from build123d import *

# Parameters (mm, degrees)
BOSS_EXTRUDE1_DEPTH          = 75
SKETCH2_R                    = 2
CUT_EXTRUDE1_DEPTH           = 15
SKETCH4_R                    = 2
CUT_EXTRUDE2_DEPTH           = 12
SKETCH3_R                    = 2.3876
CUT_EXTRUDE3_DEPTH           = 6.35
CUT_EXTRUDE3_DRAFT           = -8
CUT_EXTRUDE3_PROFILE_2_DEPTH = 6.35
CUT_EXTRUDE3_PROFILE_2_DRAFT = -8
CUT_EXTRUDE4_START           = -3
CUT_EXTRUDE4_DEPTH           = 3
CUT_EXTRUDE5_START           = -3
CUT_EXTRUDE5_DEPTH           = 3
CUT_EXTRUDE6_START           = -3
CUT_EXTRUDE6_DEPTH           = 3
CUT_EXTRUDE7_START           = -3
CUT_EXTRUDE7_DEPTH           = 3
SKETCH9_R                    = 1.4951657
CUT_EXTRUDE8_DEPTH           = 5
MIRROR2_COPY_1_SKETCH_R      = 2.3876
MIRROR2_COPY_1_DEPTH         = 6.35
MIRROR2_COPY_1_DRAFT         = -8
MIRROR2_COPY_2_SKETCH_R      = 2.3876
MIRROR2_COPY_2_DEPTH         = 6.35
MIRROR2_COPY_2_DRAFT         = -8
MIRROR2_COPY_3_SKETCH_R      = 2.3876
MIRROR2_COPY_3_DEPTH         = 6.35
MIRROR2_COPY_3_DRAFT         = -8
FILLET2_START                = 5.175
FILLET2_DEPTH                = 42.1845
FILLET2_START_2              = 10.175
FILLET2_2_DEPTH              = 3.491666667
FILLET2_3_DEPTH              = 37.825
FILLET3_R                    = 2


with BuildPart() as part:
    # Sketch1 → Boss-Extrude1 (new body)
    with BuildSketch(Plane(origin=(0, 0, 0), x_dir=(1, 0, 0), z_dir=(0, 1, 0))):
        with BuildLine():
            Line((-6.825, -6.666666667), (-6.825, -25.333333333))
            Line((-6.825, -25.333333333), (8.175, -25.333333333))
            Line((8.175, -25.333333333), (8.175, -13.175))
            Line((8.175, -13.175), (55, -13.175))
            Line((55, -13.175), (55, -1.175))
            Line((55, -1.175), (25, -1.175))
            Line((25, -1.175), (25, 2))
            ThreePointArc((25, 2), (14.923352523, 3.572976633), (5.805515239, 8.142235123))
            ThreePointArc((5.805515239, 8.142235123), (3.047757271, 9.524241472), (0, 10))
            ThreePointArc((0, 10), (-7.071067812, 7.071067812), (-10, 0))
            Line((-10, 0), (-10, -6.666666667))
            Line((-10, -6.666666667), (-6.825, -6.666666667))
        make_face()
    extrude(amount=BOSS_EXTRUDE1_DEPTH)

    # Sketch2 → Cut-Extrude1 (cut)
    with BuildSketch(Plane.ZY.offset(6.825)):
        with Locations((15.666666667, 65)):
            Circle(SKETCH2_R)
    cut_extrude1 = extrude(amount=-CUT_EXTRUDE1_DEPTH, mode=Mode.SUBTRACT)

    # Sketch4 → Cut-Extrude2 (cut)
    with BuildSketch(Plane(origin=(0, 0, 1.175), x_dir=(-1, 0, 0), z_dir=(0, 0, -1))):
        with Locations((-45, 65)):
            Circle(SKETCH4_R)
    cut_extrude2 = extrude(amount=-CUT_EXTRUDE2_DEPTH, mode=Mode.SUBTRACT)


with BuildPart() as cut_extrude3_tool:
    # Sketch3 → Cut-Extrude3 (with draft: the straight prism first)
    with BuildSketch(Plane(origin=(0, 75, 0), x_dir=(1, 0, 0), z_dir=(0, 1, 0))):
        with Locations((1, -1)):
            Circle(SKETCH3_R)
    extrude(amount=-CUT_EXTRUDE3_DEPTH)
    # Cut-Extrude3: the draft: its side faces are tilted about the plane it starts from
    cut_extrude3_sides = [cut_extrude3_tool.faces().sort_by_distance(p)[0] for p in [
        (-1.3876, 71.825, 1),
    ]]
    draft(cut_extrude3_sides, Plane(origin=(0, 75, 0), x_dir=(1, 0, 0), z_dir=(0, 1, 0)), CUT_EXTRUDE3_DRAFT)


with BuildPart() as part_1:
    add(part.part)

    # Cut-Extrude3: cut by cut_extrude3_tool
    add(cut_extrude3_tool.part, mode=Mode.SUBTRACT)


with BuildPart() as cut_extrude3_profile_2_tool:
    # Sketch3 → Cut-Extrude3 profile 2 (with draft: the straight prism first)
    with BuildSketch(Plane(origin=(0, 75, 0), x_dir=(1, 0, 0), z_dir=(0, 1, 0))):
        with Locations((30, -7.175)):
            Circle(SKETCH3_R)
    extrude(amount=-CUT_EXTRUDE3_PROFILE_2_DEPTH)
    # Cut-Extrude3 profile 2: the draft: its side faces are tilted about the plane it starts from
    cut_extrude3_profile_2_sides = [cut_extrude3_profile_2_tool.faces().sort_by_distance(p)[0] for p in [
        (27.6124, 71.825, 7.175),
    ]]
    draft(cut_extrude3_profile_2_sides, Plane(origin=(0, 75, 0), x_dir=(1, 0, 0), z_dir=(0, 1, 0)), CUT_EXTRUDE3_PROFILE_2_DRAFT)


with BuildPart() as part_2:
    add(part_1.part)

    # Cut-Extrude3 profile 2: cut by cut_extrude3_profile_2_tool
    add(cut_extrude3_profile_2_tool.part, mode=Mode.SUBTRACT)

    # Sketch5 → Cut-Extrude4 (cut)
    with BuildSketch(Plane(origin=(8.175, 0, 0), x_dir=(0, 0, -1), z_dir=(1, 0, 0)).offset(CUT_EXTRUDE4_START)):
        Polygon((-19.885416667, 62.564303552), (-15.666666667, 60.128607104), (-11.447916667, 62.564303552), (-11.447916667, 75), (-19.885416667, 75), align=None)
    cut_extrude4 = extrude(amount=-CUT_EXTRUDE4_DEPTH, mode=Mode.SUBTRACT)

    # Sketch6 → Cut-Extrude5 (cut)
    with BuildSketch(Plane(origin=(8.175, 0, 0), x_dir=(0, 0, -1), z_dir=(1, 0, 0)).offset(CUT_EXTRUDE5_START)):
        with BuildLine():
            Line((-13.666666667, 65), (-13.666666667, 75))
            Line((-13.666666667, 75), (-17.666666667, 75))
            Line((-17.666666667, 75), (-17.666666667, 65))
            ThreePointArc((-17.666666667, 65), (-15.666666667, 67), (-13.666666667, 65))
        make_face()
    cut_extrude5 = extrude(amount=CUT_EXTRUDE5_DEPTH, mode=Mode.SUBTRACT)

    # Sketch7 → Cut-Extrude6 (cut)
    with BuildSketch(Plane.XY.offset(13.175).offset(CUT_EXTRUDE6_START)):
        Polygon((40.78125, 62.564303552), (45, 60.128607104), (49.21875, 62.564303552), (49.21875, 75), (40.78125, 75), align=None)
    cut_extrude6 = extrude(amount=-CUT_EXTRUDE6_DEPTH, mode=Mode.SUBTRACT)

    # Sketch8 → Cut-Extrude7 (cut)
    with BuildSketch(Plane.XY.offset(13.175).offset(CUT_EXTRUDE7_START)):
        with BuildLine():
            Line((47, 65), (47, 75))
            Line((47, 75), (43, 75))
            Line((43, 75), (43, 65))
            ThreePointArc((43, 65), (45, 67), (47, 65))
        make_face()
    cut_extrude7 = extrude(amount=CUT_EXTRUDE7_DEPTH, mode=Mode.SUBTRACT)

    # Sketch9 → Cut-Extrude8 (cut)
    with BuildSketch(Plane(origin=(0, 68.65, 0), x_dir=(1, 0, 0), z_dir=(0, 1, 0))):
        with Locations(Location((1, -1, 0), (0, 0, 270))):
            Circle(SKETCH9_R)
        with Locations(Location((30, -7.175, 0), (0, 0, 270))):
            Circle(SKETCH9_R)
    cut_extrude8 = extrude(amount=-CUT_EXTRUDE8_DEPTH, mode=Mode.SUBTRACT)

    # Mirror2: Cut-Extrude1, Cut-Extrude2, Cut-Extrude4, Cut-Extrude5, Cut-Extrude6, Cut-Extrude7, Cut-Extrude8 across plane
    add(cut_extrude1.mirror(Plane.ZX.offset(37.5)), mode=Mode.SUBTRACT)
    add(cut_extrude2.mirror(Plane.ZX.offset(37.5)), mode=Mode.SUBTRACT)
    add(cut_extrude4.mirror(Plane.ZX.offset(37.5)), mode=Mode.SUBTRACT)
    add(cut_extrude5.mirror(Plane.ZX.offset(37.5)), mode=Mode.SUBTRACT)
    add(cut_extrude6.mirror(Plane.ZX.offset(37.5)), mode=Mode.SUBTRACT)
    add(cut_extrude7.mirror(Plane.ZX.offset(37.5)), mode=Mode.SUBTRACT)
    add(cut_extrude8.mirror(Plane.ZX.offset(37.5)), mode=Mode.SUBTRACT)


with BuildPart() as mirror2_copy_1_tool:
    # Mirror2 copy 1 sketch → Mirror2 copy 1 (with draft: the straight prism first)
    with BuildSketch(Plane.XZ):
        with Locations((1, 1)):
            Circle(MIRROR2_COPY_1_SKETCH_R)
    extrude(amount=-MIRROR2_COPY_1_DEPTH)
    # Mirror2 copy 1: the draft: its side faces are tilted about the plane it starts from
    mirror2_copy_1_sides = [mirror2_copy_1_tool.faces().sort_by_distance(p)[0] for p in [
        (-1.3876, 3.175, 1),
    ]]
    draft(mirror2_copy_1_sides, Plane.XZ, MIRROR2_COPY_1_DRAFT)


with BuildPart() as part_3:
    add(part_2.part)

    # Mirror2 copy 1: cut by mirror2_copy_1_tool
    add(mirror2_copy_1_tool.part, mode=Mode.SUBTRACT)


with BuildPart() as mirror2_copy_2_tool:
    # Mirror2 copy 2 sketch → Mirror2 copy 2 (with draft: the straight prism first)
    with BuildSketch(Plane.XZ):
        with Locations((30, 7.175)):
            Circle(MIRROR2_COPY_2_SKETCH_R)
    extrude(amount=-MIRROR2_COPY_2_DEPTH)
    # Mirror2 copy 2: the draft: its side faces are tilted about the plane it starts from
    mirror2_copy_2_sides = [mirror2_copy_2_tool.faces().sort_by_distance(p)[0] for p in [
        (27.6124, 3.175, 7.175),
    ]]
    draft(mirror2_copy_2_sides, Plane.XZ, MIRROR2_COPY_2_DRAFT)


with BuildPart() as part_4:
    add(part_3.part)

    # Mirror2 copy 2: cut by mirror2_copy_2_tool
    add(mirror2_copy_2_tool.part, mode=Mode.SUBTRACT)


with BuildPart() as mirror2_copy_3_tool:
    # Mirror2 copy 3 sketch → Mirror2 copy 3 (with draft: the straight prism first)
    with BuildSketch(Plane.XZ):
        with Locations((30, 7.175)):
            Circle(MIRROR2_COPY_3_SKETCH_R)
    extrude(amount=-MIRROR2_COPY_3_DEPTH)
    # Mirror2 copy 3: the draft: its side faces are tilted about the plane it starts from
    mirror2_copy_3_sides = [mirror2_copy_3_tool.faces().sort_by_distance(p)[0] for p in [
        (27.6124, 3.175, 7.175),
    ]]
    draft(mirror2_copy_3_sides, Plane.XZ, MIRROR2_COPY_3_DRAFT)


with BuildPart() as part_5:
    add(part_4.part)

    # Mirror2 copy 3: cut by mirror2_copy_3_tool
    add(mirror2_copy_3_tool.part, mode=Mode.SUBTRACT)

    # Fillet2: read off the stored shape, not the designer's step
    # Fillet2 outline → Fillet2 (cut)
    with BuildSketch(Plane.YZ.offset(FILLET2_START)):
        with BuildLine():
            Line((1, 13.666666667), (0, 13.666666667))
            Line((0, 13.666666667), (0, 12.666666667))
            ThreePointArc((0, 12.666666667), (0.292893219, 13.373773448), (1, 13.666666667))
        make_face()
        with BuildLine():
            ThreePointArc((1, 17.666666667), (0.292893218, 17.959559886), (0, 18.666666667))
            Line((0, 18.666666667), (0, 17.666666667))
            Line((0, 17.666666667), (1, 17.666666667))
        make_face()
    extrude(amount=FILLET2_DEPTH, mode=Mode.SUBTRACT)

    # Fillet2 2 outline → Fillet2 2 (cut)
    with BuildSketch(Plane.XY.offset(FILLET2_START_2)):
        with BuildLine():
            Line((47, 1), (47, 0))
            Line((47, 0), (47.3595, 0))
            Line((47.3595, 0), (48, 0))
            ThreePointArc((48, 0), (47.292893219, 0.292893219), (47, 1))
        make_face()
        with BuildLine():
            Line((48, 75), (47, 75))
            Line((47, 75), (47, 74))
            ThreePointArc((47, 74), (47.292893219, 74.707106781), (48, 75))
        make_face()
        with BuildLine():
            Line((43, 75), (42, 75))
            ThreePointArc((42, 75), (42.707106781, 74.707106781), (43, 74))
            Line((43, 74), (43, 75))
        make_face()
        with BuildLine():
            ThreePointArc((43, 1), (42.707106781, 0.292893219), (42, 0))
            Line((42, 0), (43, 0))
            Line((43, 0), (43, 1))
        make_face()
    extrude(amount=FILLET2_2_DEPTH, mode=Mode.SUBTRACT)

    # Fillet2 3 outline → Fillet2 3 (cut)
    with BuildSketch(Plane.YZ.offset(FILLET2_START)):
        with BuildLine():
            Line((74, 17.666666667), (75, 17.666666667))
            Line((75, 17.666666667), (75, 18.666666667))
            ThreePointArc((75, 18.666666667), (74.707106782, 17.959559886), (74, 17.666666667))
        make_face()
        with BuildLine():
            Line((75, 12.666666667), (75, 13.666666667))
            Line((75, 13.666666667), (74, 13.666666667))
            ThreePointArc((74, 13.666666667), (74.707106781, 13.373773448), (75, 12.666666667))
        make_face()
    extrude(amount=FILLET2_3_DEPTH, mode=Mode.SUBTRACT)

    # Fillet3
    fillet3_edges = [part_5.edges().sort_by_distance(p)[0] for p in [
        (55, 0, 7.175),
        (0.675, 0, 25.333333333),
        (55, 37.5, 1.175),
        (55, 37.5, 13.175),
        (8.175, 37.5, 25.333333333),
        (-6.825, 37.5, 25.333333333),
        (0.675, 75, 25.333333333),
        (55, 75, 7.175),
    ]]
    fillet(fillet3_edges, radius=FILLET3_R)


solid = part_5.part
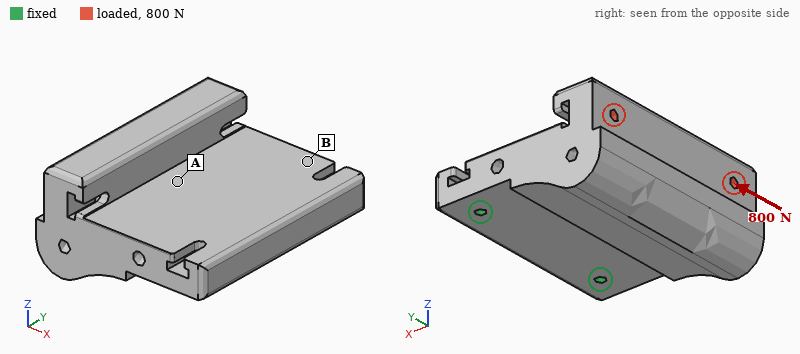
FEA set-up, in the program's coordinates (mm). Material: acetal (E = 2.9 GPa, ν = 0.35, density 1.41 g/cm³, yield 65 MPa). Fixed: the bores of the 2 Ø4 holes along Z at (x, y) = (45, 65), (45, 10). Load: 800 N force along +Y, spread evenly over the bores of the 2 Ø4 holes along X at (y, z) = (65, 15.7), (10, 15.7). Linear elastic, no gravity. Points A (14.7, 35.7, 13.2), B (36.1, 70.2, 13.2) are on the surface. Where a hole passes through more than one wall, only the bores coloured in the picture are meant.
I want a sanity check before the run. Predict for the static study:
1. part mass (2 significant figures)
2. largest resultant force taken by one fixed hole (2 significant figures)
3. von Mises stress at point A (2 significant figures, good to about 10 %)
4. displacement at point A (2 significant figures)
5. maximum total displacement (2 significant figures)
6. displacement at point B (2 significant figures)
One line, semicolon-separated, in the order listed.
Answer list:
120 g; 800 N; 3.7 MPa; 0.075 mm; 0.19 mm; 0.040 mm
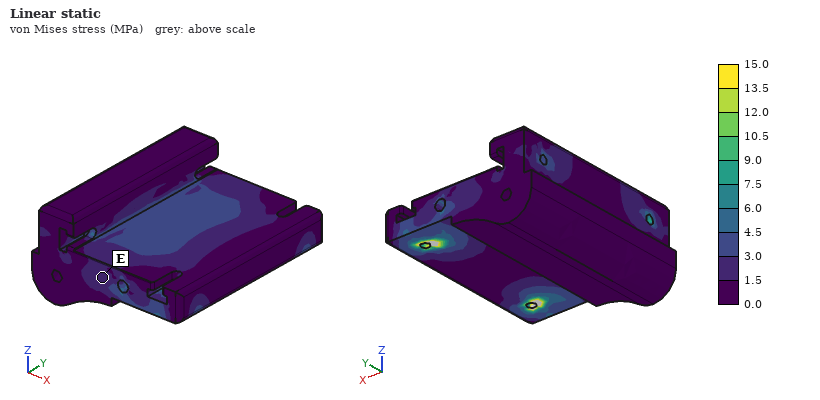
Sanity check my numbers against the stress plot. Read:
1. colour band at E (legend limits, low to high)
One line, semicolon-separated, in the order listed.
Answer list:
1.5 to 3.0 MPa
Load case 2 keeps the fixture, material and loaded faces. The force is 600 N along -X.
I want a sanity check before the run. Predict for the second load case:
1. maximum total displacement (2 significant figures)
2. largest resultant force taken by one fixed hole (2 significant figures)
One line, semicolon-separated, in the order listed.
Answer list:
0.84 mm; 300 N
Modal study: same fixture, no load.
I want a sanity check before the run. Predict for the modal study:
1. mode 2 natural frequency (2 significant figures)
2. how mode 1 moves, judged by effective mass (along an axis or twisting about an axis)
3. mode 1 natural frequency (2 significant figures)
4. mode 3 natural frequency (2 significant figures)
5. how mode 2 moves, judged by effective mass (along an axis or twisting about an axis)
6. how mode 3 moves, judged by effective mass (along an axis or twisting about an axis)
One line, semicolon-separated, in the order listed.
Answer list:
1200 Hz; along Z; 290 Hz; 1600 Hz; twisting about X; along Y
